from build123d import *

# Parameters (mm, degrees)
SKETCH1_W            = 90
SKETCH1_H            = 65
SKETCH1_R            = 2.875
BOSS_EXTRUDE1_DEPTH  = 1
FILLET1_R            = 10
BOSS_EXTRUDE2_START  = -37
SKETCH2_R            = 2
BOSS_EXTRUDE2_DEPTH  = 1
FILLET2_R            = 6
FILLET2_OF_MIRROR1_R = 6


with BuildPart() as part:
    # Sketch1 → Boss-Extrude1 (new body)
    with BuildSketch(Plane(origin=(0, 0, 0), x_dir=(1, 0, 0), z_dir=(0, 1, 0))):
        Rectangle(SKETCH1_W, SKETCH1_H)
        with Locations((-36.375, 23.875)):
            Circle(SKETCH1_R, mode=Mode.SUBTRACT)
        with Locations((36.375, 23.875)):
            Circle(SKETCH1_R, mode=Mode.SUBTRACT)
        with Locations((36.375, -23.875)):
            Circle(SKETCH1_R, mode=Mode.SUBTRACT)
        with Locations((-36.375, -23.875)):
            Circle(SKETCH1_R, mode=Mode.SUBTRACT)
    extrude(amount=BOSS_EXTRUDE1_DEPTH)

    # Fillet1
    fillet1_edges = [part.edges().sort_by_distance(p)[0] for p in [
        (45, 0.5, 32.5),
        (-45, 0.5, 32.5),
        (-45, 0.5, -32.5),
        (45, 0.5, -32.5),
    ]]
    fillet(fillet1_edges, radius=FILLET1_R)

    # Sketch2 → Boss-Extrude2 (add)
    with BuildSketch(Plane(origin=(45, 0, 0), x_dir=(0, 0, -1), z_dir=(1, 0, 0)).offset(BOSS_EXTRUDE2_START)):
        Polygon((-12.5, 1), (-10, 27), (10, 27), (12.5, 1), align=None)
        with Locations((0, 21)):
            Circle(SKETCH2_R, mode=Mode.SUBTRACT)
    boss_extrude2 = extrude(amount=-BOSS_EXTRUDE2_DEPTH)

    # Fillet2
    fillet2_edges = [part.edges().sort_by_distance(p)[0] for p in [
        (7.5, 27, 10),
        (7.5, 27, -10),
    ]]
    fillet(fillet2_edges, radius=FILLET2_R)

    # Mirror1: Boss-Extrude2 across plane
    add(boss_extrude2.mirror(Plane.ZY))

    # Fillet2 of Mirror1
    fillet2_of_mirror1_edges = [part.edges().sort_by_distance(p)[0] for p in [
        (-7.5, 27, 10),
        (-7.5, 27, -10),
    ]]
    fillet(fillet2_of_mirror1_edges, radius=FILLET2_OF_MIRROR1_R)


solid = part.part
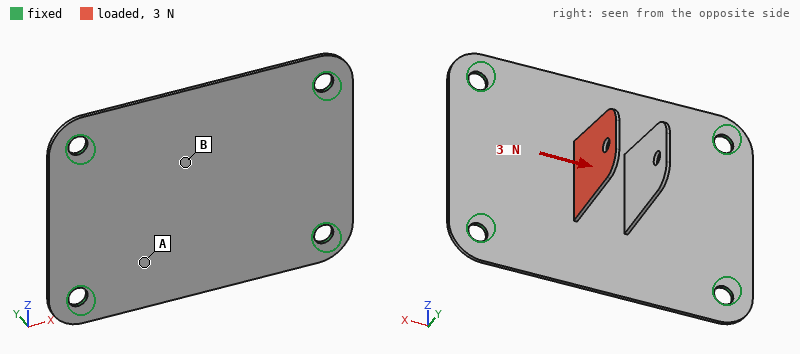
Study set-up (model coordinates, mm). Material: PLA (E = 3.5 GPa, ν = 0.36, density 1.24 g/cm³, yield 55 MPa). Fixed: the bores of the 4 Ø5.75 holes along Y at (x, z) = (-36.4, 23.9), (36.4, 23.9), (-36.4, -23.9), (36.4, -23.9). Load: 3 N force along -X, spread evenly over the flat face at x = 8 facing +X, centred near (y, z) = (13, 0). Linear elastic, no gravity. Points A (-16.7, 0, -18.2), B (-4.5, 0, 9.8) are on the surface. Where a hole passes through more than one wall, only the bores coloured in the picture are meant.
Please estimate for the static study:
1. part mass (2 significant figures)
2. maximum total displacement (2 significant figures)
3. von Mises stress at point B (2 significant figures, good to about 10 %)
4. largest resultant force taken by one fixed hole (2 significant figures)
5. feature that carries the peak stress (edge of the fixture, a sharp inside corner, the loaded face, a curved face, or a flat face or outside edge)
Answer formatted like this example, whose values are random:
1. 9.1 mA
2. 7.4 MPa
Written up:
1. 8.4 g
2. 1.2 mm
3. 1.3 MPa
4. 0.97 N
5. the loaded face
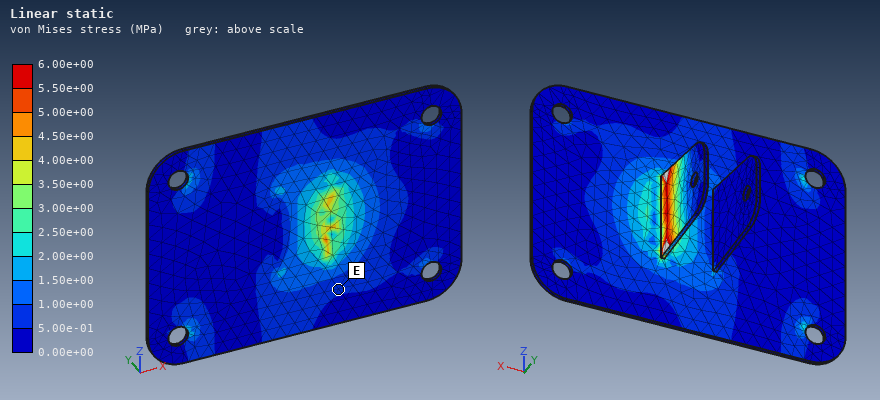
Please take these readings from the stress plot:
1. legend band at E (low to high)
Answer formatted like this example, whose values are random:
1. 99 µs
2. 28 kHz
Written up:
1. 5.00e-01 to 1.00e+00 MPa
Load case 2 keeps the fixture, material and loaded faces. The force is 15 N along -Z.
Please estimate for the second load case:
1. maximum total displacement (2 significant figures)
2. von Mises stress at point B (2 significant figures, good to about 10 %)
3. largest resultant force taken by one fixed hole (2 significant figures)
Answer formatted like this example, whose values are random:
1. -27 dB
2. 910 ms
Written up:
1. 1.1 mm
2. 2.1 MPa
3. 5.9 N
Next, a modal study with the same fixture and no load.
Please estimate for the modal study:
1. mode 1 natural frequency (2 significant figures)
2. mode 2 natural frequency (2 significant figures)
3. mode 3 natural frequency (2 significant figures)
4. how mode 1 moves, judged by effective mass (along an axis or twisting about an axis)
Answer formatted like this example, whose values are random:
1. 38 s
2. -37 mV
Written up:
1. 260 Hz
2. 380 Hz
3. 390 Hz
4. along Y
